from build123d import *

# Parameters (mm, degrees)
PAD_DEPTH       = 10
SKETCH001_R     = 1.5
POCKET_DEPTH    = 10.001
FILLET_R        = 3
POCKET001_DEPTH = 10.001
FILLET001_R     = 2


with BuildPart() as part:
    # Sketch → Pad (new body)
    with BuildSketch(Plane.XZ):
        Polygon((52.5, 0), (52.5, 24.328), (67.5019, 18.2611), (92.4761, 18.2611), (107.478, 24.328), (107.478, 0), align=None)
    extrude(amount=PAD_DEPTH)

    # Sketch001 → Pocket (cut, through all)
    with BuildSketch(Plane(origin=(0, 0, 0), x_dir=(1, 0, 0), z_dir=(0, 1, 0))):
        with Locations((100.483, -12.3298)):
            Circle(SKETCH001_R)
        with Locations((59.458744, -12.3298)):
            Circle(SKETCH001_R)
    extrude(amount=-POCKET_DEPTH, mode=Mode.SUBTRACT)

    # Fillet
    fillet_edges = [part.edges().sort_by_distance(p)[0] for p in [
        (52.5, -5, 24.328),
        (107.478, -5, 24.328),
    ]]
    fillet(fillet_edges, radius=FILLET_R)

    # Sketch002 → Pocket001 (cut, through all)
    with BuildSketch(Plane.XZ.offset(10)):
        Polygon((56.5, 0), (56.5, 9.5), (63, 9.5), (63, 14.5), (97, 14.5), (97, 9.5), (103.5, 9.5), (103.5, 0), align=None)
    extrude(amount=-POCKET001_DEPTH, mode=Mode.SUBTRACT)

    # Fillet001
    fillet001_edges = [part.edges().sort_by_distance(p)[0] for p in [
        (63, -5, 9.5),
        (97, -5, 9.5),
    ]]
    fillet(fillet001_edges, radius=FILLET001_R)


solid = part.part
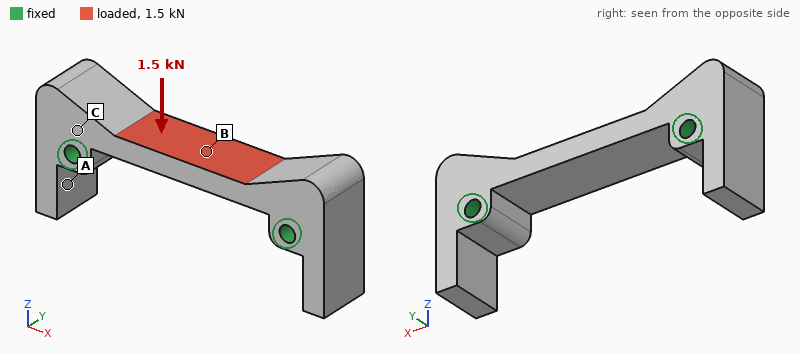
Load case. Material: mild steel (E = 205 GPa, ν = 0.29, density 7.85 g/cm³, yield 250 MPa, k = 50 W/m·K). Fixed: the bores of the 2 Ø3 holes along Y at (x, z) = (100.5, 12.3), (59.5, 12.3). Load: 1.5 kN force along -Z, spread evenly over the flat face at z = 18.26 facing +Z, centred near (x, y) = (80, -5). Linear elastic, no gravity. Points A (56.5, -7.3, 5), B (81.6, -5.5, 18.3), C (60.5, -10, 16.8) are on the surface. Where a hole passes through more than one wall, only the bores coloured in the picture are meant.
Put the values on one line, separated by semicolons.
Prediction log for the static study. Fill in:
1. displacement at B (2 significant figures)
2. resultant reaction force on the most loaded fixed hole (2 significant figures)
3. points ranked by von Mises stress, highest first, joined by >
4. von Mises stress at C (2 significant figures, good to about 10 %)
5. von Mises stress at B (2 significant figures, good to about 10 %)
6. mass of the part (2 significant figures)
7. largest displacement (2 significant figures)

27 µm; 850 N; B > C > A; 46 MPa; 120 MPa; 36 g; 29 µm
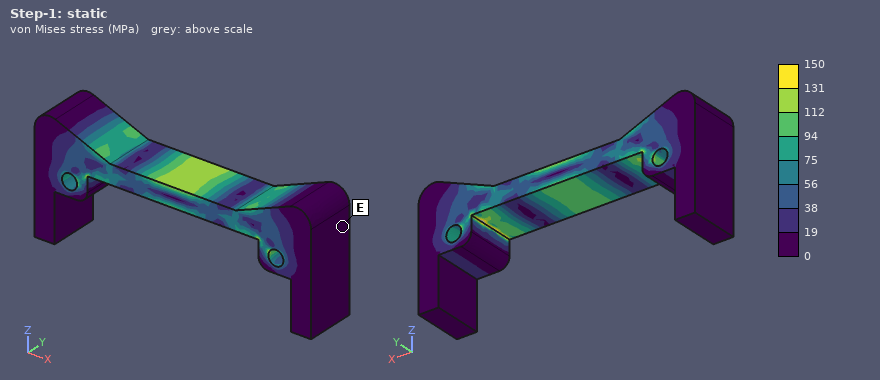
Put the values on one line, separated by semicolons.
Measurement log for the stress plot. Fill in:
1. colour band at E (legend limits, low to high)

0 to 19 MPa
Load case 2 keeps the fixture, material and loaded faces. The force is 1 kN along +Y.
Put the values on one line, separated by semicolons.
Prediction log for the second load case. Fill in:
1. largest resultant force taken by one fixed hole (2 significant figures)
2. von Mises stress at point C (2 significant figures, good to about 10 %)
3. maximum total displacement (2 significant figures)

500 N; 25 MPa; 9.0 µm
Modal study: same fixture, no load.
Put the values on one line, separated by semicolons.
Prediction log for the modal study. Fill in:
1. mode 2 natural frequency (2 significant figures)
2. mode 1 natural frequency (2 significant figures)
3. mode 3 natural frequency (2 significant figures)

19 kHz; 14 kHz; 21 kHz
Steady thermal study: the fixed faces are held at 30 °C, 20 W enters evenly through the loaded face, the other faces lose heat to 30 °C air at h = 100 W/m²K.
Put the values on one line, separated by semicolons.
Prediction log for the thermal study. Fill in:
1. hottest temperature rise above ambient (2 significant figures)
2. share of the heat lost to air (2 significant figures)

61 K; 16 %
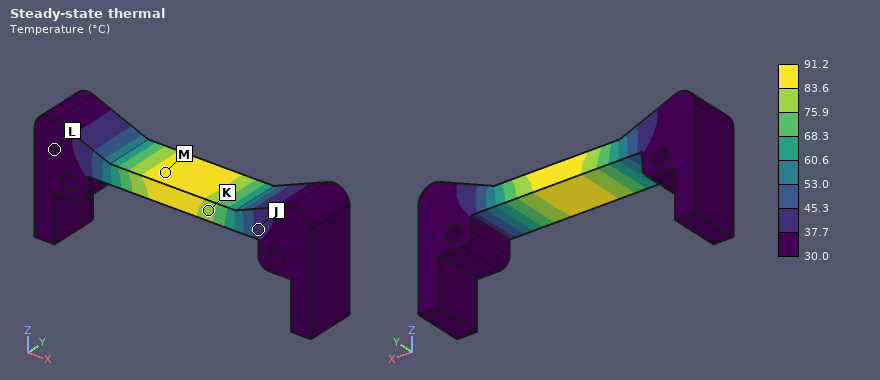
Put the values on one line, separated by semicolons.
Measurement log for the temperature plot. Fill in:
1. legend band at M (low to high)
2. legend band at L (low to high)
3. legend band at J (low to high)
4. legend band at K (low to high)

83.6 to 91.2 °C; 30.0 to 37.7 °C; 37.7 to 45.3 °C; 75.9 to 83.6 °C
